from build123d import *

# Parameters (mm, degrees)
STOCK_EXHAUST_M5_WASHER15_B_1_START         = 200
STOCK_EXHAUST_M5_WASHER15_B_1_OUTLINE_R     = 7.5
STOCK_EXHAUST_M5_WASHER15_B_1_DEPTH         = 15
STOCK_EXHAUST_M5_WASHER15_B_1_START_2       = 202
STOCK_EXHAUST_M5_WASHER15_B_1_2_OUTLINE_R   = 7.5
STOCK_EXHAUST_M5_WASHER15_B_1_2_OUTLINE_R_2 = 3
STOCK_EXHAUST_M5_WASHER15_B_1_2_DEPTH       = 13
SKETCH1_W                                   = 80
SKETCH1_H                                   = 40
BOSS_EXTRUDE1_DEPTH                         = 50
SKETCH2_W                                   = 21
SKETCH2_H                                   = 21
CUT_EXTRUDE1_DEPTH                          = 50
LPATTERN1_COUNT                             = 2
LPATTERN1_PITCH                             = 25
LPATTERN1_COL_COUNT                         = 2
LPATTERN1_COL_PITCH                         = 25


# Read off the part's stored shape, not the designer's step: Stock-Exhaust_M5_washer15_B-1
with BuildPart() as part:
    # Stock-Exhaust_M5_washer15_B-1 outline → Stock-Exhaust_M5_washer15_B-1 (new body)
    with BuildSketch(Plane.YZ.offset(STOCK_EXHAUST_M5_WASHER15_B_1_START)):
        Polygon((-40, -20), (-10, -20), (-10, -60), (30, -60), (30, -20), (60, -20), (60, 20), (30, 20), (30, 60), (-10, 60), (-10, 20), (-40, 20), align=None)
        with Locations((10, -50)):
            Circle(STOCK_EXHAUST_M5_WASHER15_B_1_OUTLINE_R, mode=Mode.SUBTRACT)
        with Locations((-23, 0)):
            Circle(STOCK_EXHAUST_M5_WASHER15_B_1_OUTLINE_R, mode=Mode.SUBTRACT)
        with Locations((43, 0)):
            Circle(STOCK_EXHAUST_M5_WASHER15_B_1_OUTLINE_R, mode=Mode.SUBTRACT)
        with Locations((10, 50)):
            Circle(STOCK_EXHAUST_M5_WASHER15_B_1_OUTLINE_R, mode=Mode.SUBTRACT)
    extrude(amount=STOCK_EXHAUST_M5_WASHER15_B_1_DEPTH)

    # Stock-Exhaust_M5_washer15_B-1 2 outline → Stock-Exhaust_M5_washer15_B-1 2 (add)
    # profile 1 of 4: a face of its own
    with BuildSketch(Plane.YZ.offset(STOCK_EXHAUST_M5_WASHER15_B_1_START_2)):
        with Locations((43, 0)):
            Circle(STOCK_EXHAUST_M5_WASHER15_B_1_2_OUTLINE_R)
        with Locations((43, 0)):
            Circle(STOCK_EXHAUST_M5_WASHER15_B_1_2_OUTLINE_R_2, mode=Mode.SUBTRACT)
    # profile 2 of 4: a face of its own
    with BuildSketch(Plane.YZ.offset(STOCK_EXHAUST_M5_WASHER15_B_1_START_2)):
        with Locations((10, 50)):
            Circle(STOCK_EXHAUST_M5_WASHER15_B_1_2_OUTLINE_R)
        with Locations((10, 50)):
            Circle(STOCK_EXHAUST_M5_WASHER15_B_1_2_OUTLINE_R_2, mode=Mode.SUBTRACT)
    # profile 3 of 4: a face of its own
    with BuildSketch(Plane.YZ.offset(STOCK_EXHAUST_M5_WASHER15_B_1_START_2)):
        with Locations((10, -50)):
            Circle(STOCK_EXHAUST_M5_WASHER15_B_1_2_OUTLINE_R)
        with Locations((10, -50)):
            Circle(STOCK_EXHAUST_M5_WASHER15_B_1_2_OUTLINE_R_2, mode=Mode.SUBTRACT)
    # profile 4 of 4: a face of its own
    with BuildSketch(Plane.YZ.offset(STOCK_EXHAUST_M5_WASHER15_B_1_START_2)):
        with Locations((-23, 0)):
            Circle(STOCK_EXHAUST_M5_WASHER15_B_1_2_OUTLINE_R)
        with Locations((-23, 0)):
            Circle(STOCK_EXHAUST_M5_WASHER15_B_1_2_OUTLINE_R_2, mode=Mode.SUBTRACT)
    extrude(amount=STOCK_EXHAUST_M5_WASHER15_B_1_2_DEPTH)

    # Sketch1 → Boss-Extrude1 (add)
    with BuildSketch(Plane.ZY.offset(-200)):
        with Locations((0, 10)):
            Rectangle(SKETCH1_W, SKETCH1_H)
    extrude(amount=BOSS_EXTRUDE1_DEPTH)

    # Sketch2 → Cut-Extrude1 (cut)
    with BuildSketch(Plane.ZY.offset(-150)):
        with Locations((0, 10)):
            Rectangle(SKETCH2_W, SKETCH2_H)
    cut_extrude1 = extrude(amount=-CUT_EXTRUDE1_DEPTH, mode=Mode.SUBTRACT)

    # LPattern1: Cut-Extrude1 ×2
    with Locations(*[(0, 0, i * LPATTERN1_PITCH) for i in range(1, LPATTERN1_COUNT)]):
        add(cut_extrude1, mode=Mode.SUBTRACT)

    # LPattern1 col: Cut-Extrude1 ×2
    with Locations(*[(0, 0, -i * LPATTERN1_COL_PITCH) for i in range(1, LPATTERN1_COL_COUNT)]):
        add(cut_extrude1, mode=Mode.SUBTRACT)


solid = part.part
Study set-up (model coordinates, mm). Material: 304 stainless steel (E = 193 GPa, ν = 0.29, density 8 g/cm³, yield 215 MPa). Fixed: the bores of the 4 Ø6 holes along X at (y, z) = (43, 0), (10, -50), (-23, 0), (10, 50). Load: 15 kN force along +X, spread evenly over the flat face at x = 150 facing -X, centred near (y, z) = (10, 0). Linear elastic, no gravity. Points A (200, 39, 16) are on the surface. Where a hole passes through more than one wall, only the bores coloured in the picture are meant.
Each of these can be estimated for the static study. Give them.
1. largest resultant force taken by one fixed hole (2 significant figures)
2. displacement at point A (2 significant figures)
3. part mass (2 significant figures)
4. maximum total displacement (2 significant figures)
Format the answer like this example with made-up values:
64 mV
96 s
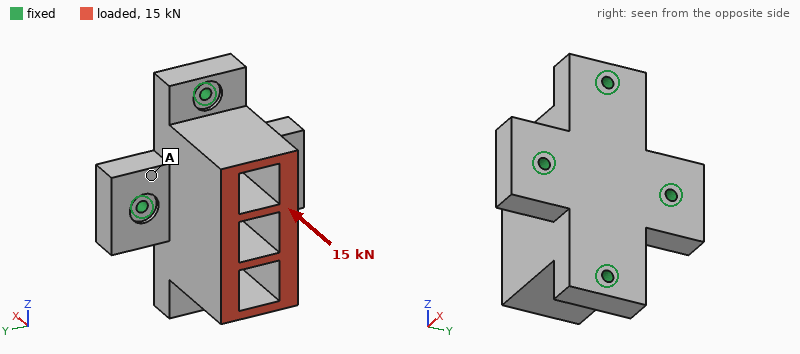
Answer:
4.0 kN
2.4 µm
1.6 kg
6.0 µm
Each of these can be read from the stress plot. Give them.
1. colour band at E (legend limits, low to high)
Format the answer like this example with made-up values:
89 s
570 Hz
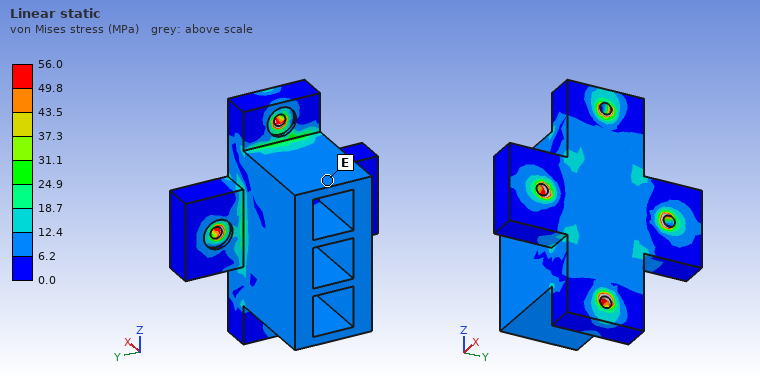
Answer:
6.2 to 12.4 MPa
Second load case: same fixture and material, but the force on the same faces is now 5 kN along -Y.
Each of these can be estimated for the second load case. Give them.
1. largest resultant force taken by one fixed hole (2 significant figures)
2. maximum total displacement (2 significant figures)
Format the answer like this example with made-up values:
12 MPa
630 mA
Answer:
4.6 kN
20 µm
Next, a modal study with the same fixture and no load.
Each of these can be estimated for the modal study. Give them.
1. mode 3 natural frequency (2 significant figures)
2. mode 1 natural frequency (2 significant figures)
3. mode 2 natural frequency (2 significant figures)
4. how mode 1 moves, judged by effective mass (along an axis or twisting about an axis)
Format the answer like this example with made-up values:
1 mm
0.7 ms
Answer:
6700 Hz
4800 Hz
6600 Hz
along Y
